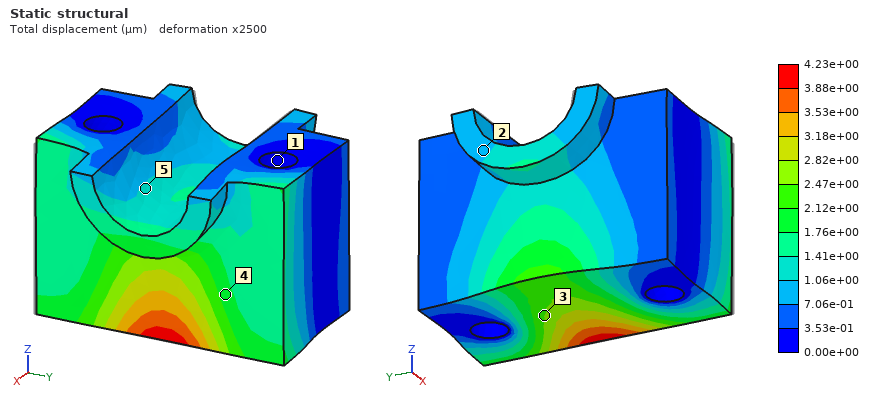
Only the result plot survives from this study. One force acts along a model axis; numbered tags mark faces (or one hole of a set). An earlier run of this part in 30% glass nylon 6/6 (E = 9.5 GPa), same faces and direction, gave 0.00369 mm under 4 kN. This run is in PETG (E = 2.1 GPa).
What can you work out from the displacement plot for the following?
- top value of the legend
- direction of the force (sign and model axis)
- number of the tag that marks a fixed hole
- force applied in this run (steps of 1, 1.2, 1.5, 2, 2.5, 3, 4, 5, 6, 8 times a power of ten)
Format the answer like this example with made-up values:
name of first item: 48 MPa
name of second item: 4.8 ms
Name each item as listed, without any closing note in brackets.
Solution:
top value of the legend: 4.23e+00 µm
direction of the force: -X
number of the tag that marks a fixed hole: 1
force applied in this run: 1 kN
